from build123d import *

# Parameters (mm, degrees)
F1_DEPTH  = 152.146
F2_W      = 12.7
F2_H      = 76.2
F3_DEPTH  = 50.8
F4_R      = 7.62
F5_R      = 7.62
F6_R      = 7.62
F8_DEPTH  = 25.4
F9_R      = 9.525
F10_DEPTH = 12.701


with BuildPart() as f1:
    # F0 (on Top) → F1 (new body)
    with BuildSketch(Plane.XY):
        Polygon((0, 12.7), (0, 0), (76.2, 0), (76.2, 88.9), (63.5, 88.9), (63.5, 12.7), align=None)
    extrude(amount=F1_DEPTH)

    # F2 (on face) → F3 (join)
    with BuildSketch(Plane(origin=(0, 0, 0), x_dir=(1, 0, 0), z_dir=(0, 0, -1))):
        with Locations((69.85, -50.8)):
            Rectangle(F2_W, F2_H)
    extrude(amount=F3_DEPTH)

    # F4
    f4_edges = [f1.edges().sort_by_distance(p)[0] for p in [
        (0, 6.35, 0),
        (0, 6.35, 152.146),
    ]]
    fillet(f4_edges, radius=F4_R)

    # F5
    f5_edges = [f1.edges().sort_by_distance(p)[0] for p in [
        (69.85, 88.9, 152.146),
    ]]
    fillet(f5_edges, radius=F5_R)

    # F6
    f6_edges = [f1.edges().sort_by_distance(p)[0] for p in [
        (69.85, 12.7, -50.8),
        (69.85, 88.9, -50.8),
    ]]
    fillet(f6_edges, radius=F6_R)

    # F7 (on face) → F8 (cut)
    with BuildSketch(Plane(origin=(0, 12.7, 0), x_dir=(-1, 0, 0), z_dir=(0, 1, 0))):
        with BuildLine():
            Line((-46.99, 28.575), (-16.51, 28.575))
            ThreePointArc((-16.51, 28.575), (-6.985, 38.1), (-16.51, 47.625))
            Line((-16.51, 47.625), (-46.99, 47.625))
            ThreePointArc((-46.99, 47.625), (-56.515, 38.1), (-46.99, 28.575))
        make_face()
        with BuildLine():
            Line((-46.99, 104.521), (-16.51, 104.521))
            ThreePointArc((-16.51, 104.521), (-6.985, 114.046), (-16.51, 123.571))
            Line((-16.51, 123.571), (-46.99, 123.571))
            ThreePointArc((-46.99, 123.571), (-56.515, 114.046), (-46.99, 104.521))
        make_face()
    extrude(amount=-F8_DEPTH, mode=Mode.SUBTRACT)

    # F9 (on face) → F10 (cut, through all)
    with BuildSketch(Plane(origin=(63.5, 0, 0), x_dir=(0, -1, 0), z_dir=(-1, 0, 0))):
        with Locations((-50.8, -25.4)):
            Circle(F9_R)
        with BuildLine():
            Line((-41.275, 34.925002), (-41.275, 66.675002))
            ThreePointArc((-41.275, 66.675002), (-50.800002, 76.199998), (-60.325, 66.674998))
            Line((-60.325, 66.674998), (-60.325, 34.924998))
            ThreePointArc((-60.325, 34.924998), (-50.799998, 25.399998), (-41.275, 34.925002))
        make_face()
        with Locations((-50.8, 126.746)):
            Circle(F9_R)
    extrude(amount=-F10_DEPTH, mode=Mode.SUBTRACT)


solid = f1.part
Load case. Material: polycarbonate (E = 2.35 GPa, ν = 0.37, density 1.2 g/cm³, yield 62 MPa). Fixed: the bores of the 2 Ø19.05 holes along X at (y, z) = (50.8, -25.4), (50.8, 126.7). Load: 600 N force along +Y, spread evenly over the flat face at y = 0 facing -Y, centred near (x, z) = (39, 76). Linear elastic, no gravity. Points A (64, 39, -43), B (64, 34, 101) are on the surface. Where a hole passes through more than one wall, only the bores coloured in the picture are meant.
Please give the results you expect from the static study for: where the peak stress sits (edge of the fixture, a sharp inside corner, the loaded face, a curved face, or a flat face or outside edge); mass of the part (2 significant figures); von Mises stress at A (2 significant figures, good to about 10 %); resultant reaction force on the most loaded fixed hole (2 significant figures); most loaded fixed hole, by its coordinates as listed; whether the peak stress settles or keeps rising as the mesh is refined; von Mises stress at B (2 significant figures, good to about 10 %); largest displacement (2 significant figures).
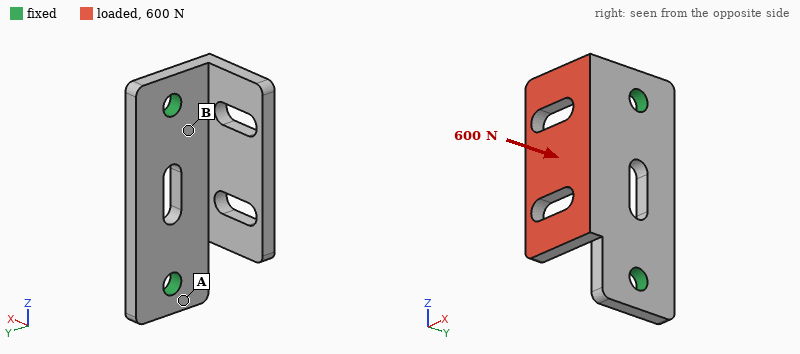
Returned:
edge of the fixture
360 g
1.3 MPa
410 N
(50.8, 126.7)
keeps rising
4.4 MPa
1.4 mm
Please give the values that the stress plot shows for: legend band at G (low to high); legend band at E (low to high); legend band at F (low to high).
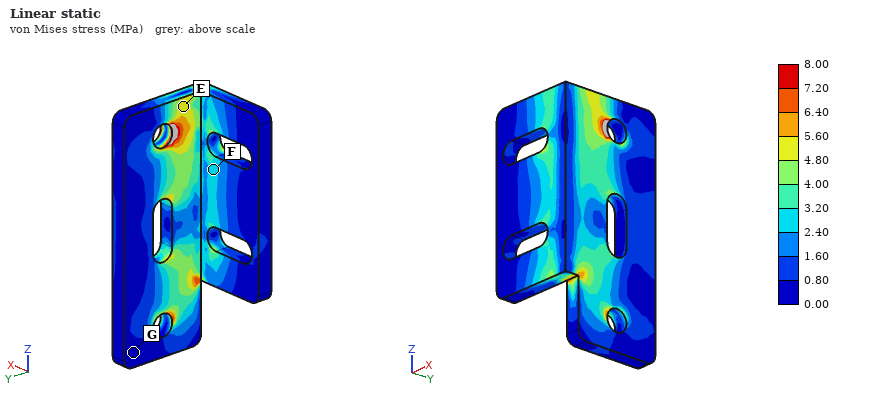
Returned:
0.00 to 0.80 MPa
4.80 to 5.60 MPa
2.40 to 3.20 MPa
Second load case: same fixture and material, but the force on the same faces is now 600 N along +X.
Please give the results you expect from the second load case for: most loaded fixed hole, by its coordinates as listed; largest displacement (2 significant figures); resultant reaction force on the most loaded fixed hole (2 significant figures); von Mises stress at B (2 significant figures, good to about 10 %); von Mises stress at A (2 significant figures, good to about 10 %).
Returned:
(50.8, 126.7)
1.2 mm
390 N
4.1 MPa
2.0 MPa
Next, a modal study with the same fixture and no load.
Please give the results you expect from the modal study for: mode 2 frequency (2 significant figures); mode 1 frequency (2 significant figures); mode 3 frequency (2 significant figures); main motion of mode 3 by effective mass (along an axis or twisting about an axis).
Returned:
540 Hz
300 Hz
700 Hz
along X
